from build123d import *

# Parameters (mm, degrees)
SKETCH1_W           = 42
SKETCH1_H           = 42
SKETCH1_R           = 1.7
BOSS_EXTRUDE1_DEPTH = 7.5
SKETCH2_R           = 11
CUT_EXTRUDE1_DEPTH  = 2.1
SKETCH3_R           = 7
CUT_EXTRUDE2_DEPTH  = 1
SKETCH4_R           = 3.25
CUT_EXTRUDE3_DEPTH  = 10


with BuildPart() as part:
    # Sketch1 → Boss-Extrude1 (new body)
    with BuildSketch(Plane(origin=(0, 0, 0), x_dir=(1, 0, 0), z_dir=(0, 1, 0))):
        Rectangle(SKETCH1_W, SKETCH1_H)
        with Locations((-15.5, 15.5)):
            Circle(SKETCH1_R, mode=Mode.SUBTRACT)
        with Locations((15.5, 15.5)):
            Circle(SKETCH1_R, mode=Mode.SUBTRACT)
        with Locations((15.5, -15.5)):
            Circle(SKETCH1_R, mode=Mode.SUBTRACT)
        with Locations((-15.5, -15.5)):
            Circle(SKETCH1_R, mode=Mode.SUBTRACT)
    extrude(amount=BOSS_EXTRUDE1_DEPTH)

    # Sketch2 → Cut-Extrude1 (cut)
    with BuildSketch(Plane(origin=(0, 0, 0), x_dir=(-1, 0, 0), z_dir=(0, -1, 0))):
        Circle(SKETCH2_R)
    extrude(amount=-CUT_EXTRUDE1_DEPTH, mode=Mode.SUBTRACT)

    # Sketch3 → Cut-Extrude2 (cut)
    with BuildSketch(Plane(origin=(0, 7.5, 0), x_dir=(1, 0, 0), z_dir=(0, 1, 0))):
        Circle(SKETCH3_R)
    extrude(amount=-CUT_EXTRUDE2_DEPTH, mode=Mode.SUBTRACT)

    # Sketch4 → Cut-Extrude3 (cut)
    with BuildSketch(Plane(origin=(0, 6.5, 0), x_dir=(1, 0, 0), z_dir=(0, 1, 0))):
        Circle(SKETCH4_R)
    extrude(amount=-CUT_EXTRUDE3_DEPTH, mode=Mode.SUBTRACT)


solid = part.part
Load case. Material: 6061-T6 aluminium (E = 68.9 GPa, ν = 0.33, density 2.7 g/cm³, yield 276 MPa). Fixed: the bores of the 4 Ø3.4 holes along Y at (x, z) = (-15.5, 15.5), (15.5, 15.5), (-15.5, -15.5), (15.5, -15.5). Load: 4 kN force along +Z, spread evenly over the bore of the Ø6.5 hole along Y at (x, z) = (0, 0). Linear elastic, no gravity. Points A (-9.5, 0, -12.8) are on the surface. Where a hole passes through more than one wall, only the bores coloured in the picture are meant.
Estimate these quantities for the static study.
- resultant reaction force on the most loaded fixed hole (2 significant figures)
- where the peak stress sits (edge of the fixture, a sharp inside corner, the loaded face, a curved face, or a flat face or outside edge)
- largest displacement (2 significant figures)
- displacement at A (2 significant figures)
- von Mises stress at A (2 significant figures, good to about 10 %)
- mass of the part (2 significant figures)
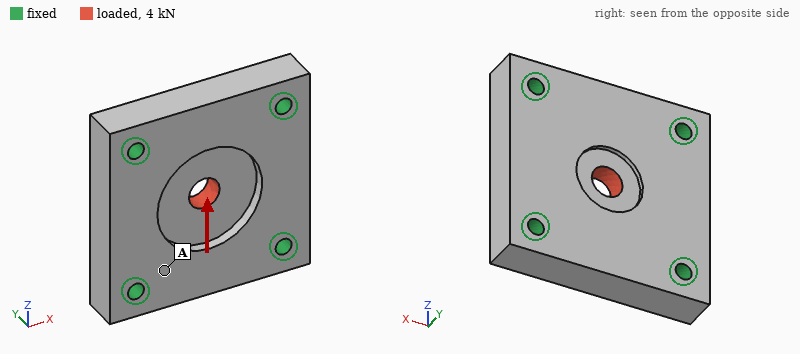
1.1 kN
the loaded face
7.8 µm
1.9 µm
11 MPa
32 g
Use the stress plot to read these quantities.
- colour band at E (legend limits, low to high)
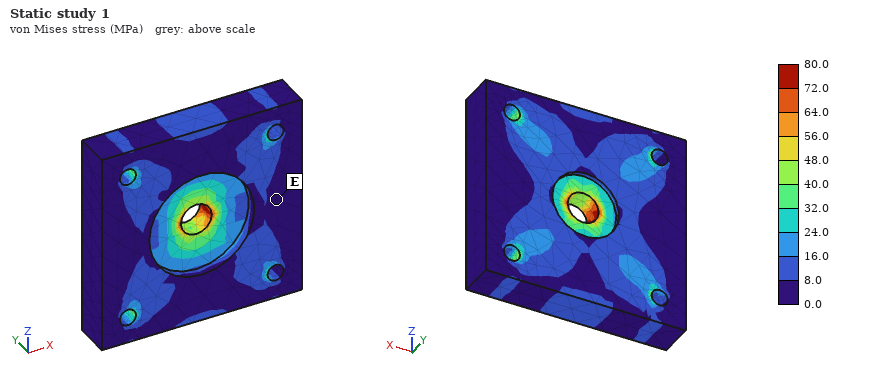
0.0 to 8.0 MPa
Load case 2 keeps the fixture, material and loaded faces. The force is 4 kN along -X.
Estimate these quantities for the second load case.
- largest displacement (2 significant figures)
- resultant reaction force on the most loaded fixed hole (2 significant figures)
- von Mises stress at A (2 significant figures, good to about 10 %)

7.8 µm
1.1 kN
12 MPa
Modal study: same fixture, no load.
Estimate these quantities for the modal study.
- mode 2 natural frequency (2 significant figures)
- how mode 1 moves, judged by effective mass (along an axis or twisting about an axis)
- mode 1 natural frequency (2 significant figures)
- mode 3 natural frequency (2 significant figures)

32 kHz
along Y
22 kHz
32 kHz
